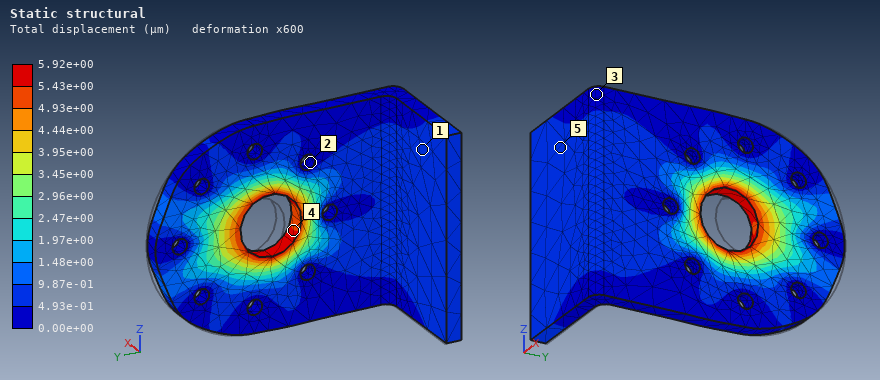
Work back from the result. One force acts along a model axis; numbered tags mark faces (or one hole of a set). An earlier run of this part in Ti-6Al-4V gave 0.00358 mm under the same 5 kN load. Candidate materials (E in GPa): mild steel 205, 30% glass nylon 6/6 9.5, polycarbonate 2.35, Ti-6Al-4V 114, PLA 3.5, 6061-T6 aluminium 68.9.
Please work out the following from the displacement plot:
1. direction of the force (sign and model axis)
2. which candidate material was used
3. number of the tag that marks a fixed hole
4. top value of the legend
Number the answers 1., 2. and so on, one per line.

1. -Y
2. 6061-T6 aluminium
3. 2
4. 5.92e+00 µm
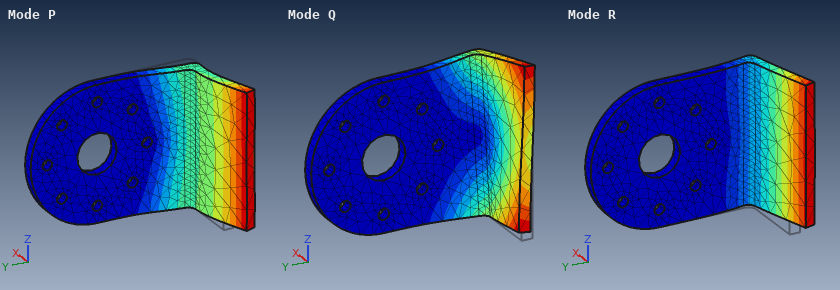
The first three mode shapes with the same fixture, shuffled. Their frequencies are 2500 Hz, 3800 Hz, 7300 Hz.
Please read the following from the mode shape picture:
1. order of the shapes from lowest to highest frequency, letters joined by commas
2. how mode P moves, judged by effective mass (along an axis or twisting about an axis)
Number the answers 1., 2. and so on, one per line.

1. R, Q, P
2. along X
